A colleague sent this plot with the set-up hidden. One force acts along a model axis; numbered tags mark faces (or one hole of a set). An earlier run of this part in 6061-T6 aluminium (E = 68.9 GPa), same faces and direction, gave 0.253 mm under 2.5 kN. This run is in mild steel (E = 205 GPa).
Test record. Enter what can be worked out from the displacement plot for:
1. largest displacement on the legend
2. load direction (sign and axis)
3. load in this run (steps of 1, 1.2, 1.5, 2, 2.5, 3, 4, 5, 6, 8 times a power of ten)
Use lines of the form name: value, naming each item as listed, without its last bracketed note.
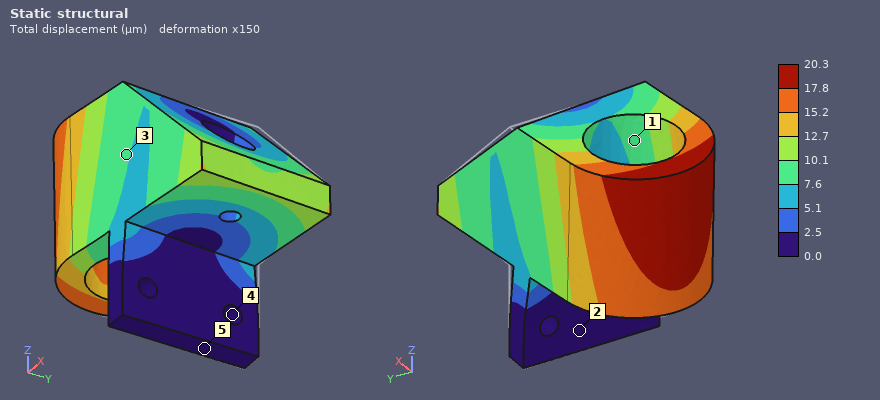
largest displacement on the legend: 20.3 µm
load direction: -Y
load in this run: 600 N
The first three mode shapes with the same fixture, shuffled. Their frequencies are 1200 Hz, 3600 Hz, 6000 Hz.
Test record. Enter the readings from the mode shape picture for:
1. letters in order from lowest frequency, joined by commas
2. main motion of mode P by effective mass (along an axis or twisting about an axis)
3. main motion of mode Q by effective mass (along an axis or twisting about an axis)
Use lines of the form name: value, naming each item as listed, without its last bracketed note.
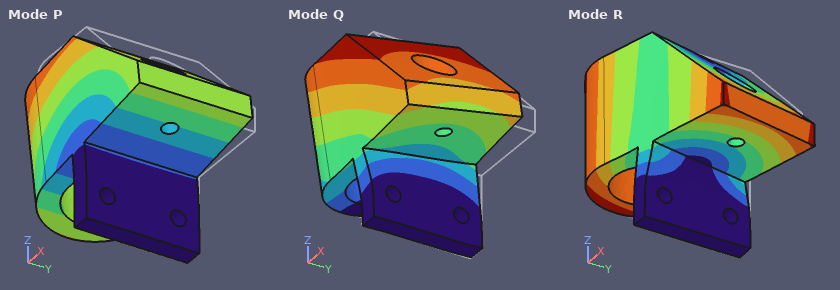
letters in order from lowest frequency, joined by commas: P, R, Q
main motion of mode P by effective mass: along X
main motion of mode Q by effective mass: along Y
